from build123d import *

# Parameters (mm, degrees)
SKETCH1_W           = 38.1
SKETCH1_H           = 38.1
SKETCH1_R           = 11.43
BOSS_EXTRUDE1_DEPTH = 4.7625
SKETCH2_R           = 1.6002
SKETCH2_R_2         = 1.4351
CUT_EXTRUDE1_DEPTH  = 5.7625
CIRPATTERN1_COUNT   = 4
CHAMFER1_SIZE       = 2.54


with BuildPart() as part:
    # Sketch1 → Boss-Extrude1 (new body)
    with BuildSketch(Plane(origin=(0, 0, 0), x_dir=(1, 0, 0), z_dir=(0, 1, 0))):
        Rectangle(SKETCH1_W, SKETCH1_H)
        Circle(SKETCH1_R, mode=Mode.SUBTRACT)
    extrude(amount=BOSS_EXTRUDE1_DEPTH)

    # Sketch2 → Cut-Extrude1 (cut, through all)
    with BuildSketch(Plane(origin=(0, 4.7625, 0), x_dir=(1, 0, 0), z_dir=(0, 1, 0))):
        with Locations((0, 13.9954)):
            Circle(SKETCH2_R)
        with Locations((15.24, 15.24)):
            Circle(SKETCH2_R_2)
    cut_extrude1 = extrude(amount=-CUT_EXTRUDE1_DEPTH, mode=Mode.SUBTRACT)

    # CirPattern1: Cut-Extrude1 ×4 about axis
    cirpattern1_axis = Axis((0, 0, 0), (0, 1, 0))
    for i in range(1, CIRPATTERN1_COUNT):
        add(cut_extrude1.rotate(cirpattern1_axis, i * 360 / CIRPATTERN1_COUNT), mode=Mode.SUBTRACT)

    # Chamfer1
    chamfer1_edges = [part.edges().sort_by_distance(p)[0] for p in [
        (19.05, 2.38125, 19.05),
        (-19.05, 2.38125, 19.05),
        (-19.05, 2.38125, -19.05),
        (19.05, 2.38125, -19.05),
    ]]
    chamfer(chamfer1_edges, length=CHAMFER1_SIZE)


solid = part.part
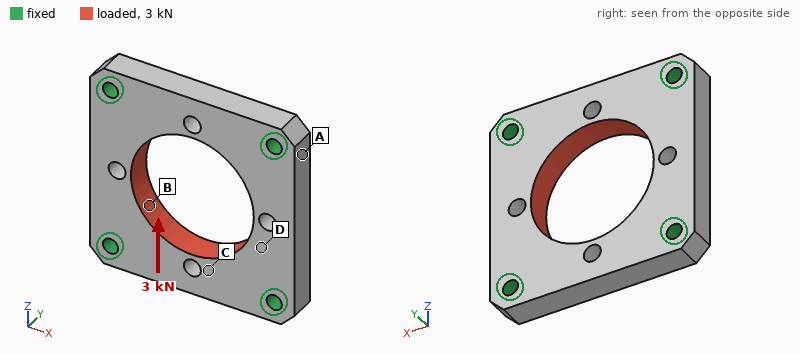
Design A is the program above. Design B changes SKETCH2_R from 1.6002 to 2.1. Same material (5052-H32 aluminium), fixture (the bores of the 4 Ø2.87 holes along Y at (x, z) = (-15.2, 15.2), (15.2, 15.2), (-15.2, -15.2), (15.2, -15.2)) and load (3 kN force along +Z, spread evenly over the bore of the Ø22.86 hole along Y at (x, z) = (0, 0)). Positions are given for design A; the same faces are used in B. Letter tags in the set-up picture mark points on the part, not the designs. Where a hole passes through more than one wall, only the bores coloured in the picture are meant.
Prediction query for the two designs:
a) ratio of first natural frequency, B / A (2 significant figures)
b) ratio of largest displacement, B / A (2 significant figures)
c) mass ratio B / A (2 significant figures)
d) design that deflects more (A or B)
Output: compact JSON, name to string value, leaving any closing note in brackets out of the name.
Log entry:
{"ratio of first natural frequency, B / A": "1.0", "ratio of largest displacement, B / A": "1.3", "mass ratio B / A": "0.98", "design that deflects more": "B"}
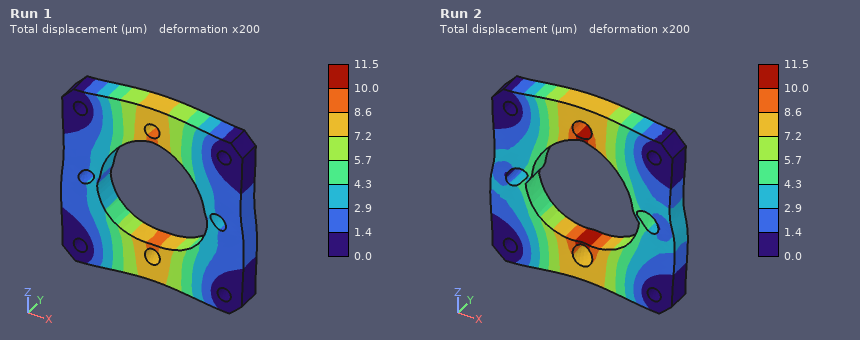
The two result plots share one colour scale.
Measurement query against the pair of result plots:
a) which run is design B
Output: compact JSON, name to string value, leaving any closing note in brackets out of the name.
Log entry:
{"which run is design B": "Run 2"}
